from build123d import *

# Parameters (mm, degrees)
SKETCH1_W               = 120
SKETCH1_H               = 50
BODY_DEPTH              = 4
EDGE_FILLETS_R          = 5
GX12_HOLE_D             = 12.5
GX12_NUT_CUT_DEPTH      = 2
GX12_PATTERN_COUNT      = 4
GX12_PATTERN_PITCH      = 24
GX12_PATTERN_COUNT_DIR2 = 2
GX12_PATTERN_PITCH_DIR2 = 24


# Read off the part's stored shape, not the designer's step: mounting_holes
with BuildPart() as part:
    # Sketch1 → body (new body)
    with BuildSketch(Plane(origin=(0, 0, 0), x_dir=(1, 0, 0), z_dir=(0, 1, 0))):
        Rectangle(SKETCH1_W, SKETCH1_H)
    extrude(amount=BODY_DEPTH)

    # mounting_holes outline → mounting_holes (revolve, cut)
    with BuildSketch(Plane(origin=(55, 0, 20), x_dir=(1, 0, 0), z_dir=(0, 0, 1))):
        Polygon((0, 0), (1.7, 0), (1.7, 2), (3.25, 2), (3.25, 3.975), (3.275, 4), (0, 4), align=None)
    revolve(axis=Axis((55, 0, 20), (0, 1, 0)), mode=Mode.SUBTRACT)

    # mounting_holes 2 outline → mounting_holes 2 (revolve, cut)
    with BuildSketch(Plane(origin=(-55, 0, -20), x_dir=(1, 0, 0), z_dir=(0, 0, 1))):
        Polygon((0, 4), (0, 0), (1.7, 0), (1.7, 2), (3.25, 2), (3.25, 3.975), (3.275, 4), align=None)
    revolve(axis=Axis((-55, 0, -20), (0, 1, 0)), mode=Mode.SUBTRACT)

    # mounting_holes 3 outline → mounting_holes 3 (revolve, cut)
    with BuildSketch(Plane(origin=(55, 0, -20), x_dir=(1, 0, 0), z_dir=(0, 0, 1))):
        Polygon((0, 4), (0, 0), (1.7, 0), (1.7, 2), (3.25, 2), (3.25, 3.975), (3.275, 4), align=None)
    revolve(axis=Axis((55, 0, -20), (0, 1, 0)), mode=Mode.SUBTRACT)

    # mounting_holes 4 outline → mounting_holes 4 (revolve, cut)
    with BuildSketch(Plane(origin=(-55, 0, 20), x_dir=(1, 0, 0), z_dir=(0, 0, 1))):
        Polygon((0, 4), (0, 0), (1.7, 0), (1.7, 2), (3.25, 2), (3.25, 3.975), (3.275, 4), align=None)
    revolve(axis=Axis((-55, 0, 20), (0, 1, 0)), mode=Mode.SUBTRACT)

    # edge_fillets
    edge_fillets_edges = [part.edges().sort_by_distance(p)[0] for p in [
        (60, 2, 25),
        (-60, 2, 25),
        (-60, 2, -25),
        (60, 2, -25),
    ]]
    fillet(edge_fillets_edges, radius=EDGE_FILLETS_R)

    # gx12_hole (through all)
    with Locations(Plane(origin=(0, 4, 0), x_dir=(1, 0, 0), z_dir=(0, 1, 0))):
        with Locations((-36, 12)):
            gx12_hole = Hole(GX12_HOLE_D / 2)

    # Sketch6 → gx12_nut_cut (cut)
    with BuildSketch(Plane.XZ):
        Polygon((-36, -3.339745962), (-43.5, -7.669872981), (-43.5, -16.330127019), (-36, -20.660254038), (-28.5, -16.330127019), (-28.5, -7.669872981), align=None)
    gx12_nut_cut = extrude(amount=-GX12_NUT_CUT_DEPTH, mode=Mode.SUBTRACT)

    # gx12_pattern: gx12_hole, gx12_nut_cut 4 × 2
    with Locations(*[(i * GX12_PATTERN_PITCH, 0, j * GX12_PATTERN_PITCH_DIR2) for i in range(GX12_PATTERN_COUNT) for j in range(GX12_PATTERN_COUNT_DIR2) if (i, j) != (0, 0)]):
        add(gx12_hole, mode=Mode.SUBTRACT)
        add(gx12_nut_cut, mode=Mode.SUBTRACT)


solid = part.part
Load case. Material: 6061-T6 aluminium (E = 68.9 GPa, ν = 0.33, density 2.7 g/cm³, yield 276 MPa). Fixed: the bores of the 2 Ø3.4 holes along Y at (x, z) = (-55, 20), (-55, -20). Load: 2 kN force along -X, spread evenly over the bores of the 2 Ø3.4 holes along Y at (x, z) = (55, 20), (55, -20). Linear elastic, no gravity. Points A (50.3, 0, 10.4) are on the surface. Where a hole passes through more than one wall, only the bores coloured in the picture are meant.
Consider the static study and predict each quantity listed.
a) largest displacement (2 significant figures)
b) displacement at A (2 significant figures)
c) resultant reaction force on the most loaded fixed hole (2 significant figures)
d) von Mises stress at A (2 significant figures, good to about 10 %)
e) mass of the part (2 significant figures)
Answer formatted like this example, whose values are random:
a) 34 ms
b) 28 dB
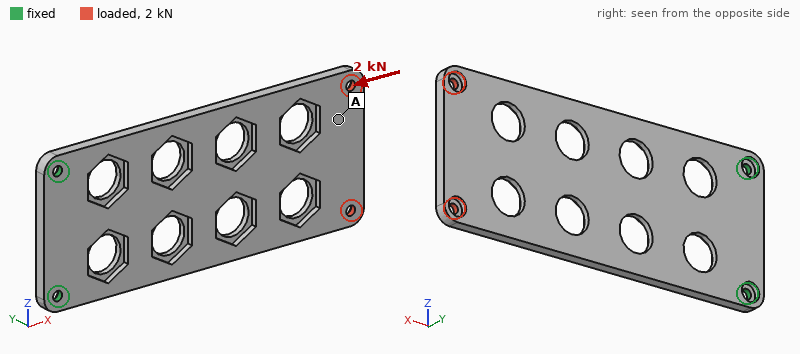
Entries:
a) 1.4 mm
b) 1.1 mm
c) 1.0 kN
d) 22 MPa
e) 50 g
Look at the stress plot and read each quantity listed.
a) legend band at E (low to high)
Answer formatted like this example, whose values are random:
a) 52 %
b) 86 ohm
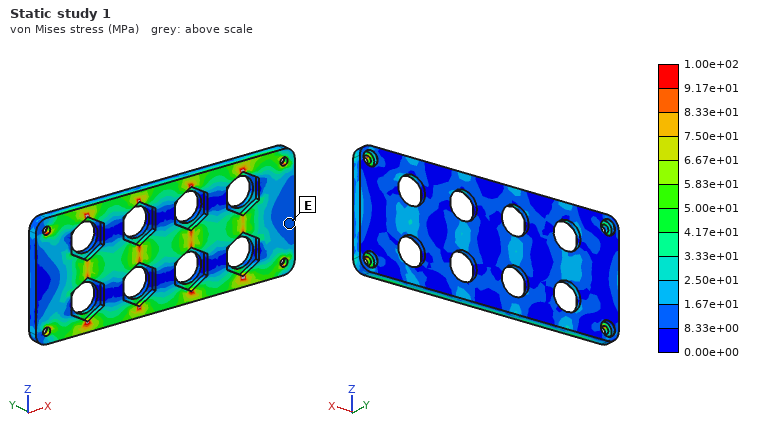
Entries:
a) 8.33e+00 to 1.67e+01 MPa
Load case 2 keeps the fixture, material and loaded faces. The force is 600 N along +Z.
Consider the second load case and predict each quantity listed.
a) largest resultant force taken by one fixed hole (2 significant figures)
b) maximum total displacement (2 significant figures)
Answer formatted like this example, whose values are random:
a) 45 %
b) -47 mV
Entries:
a) 1.6 kN
b) 0.28 mm
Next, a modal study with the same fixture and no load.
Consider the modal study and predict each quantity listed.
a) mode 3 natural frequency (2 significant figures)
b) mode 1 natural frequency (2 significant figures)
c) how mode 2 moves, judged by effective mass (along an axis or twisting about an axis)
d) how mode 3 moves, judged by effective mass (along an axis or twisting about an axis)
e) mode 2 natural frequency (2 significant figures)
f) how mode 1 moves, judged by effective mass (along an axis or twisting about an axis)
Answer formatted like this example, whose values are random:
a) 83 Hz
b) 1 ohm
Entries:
a) 1200 Hz
b) 190 Hz
c) twisting about X
d) along Y
e) 1000 Hz
f) along Y
